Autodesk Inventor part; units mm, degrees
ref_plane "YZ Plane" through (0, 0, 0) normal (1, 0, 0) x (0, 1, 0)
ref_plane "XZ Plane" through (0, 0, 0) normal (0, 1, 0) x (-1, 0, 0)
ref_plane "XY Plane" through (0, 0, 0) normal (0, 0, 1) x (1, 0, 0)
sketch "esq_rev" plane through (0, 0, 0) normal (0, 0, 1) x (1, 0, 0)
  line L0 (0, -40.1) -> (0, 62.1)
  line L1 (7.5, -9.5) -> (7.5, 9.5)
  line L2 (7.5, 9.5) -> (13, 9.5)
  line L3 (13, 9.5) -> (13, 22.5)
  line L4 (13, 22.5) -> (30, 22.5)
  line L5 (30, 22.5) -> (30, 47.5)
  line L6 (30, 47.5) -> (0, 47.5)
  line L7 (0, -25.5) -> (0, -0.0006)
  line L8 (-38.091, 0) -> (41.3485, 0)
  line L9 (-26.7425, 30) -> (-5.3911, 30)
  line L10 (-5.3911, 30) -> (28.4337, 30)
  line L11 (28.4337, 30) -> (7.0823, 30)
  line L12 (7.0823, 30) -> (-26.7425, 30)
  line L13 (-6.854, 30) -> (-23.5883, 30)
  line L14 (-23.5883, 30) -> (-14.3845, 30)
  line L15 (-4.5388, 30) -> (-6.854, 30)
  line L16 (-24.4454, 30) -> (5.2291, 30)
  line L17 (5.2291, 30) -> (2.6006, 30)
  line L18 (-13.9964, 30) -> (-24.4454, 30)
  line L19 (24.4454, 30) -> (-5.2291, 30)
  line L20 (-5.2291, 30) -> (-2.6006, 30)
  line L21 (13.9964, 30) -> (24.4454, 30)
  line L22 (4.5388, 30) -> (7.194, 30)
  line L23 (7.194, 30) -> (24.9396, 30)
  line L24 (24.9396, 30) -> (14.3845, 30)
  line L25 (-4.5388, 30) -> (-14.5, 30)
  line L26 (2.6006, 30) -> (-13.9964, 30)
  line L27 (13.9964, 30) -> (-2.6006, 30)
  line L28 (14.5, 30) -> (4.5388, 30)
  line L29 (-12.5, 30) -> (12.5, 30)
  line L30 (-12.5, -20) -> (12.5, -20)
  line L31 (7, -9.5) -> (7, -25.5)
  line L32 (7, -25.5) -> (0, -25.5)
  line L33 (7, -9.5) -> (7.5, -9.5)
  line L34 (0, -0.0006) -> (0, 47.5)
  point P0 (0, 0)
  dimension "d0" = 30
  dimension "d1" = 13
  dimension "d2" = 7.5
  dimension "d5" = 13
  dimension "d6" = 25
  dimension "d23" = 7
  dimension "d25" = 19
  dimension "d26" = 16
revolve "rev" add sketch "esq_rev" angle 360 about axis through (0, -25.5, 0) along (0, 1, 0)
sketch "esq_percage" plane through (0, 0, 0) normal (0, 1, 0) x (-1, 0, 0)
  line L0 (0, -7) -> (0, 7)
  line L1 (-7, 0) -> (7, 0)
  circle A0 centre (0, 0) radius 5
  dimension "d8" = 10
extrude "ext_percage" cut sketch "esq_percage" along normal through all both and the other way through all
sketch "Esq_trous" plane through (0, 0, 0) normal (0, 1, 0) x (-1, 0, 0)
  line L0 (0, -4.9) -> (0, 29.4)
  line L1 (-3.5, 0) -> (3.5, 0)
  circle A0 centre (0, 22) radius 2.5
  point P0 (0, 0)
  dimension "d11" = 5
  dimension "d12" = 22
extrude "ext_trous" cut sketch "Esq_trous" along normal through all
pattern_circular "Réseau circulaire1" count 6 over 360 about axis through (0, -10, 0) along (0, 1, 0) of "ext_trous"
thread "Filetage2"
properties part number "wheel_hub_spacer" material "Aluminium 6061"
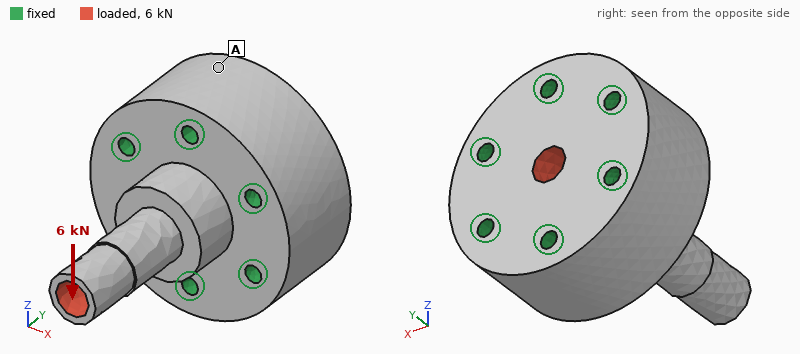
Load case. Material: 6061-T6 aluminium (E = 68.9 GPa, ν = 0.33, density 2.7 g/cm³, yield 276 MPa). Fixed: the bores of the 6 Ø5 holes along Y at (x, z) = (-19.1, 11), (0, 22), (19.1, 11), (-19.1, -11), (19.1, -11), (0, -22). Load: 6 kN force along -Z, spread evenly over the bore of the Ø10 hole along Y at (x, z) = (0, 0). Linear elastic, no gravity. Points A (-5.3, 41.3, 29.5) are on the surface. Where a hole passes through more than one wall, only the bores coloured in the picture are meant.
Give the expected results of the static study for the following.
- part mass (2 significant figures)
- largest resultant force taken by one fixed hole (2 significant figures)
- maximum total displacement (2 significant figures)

200 g
2.7 kN
0.23 mm
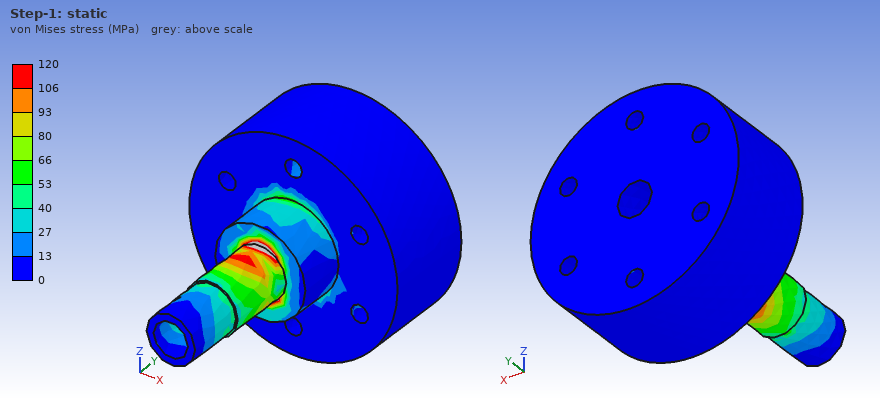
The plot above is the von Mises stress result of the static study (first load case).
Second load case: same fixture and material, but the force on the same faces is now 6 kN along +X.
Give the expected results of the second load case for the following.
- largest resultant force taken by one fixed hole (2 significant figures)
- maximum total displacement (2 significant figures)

2.4 kN
0.22 mm
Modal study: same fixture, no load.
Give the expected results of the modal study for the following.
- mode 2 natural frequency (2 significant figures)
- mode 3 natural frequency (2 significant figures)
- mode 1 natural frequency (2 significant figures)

7900 Hz
22 kHz
7900 Hz
